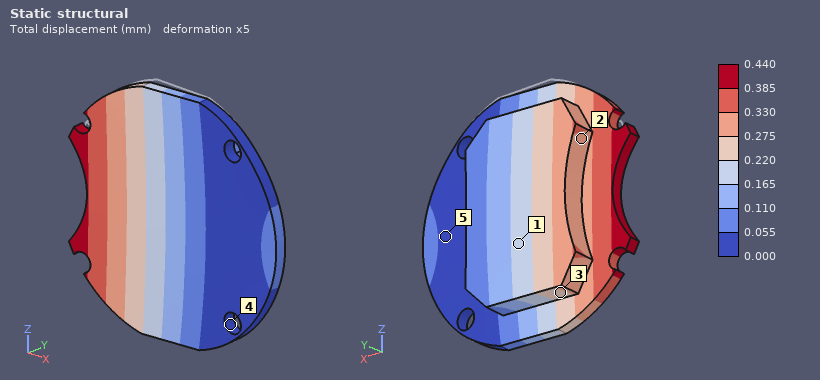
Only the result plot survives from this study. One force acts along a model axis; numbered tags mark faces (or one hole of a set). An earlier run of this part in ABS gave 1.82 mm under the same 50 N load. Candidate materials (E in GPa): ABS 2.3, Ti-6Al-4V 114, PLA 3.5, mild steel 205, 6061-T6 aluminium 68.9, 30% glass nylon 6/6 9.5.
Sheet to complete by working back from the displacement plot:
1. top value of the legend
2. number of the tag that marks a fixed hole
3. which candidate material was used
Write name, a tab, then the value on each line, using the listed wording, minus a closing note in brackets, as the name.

top value of the legend	0.440 mm
number of the tag that marks a fixed hole	4
which candidate material was used	30% glass nylon 6/6
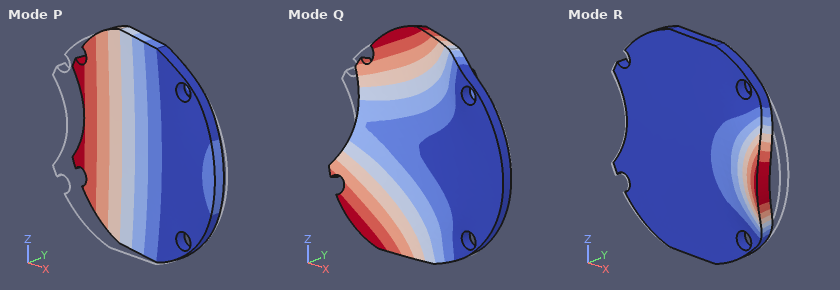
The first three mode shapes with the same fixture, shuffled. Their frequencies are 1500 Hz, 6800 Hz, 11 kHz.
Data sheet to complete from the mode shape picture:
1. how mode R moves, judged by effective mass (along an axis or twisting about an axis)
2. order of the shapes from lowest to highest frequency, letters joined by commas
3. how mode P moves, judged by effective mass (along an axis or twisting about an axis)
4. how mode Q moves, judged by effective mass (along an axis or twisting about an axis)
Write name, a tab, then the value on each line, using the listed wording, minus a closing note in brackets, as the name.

how mode R moves, judged by effective mass	along Y
order of the shapes from lowest to highest frequency, letters joined by commas	P, Q, R
how mode P moves, judged by effective mass	along Y
how mode Q moves, judged by effective mass	twisting about X
